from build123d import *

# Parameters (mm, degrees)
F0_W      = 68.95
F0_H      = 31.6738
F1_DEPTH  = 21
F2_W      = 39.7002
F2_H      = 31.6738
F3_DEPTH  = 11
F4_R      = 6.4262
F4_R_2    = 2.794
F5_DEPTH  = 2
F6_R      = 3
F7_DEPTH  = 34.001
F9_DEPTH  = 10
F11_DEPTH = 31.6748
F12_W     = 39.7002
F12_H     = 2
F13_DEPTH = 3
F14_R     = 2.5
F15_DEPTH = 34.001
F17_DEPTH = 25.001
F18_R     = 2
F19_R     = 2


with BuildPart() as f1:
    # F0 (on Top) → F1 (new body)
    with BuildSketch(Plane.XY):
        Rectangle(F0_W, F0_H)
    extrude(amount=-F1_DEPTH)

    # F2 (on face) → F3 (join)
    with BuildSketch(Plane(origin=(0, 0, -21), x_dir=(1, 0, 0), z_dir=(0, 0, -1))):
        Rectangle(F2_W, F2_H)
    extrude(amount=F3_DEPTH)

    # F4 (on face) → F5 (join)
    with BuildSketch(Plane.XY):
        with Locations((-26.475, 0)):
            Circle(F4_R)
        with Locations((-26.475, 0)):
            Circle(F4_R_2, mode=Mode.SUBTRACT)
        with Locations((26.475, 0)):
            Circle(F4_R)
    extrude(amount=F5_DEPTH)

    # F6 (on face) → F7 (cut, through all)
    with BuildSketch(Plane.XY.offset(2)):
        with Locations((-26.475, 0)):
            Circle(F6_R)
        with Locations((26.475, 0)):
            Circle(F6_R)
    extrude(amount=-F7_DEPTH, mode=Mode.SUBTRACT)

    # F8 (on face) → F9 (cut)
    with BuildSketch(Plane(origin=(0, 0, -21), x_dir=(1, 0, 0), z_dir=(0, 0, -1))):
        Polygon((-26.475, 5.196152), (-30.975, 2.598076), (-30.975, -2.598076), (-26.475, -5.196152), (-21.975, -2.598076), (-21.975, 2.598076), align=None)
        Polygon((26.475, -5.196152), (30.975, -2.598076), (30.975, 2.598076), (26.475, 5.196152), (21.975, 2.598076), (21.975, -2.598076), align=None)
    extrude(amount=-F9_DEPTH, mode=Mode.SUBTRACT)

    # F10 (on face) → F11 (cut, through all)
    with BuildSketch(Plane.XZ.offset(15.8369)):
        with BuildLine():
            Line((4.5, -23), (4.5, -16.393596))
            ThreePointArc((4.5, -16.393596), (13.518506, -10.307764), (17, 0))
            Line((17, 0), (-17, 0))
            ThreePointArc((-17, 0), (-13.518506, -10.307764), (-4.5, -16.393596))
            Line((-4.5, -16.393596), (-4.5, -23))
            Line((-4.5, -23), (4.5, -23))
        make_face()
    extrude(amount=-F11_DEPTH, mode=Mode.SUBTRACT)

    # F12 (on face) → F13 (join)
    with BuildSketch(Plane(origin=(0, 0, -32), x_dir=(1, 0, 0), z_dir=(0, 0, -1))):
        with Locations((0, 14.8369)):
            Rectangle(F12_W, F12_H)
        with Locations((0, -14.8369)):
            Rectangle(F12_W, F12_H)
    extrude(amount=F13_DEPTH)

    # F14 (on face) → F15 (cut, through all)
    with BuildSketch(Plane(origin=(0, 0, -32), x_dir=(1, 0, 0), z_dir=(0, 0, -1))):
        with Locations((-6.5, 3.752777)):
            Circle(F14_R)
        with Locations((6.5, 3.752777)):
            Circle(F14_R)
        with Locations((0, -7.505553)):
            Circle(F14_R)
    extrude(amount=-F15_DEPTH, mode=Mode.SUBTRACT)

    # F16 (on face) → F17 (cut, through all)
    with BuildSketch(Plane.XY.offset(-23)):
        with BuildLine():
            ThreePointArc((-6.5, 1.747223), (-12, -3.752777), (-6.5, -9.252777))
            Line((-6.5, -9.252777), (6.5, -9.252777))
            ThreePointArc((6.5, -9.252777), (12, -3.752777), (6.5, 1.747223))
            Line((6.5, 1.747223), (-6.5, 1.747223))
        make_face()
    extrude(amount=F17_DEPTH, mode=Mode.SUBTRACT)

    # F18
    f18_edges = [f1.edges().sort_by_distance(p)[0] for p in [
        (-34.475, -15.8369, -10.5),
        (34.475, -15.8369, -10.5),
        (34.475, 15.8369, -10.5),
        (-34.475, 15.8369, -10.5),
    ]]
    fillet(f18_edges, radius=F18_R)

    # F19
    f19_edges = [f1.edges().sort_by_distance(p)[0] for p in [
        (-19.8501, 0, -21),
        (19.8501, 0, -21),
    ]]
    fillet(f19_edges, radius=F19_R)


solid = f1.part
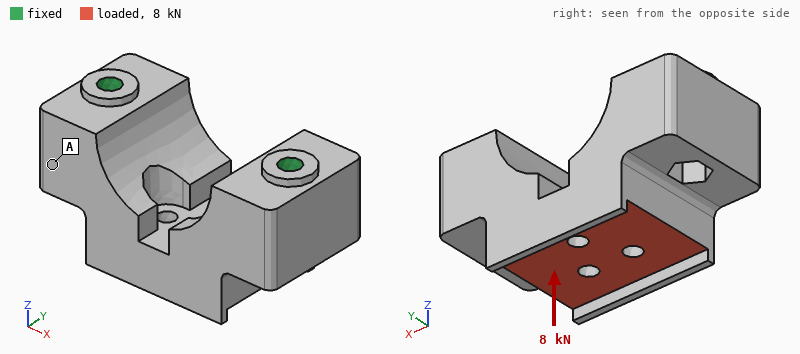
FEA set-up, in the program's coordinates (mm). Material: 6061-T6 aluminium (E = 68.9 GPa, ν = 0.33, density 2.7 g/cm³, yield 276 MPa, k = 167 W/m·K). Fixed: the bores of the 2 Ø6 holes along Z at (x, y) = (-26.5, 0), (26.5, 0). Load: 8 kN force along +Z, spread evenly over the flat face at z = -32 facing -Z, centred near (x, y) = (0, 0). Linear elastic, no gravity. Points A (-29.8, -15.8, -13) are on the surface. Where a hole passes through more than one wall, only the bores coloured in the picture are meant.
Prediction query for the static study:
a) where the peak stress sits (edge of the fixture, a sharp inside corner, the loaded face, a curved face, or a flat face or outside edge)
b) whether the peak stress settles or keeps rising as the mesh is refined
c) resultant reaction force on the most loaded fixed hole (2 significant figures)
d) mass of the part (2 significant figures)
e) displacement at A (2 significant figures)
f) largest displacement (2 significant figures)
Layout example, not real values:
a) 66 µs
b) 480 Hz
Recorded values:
a) edge of the fixture
b) keeps rising
c) 4.6 kN
d) 110 g
e) 2.7 µm
f) 12 µm
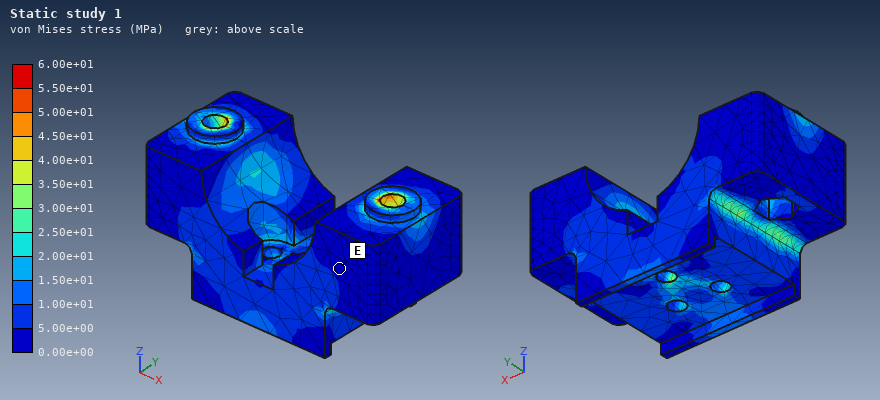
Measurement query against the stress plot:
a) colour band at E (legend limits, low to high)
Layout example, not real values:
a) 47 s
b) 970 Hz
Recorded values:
a) 0.00e+00 to 5.00e+00 MPa
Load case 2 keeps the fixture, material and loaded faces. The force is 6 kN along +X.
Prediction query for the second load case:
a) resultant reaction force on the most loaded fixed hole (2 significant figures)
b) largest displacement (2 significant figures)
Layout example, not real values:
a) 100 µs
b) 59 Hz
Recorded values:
a) 3.9 kN
b) 16 µm
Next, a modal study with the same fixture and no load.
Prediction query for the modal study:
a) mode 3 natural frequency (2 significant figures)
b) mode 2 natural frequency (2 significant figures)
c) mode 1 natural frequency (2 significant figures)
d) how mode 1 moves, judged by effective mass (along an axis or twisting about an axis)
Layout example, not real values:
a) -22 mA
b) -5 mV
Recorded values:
a) 15 kHz
b) 15 kHz
c) 7700 Hz
d) along Y
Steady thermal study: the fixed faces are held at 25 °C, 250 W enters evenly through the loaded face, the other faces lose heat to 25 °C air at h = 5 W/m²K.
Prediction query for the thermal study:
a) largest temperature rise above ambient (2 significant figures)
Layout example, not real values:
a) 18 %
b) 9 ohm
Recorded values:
a) 62 K
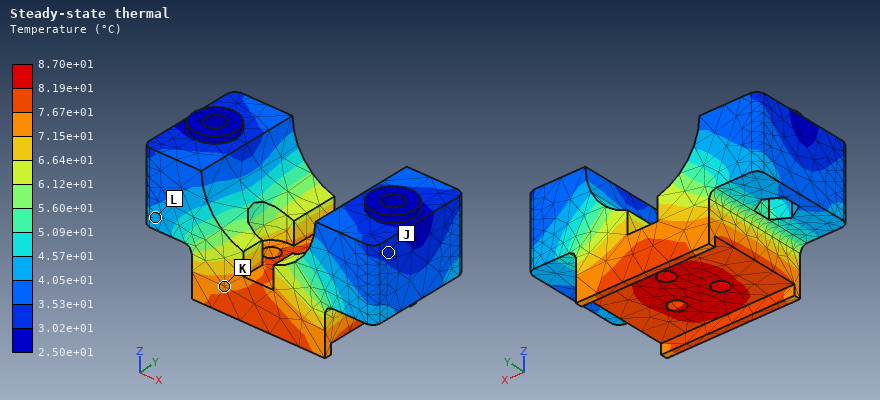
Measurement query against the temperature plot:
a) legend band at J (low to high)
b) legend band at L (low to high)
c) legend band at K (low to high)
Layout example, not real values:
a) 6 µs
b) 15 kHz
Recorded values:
a) 3.02e+01 to 3.53e+01 °C
b) 4.05e+01 to 4.57e+01 °C
c) 7.15e+01 to 7.67e+01 °C
